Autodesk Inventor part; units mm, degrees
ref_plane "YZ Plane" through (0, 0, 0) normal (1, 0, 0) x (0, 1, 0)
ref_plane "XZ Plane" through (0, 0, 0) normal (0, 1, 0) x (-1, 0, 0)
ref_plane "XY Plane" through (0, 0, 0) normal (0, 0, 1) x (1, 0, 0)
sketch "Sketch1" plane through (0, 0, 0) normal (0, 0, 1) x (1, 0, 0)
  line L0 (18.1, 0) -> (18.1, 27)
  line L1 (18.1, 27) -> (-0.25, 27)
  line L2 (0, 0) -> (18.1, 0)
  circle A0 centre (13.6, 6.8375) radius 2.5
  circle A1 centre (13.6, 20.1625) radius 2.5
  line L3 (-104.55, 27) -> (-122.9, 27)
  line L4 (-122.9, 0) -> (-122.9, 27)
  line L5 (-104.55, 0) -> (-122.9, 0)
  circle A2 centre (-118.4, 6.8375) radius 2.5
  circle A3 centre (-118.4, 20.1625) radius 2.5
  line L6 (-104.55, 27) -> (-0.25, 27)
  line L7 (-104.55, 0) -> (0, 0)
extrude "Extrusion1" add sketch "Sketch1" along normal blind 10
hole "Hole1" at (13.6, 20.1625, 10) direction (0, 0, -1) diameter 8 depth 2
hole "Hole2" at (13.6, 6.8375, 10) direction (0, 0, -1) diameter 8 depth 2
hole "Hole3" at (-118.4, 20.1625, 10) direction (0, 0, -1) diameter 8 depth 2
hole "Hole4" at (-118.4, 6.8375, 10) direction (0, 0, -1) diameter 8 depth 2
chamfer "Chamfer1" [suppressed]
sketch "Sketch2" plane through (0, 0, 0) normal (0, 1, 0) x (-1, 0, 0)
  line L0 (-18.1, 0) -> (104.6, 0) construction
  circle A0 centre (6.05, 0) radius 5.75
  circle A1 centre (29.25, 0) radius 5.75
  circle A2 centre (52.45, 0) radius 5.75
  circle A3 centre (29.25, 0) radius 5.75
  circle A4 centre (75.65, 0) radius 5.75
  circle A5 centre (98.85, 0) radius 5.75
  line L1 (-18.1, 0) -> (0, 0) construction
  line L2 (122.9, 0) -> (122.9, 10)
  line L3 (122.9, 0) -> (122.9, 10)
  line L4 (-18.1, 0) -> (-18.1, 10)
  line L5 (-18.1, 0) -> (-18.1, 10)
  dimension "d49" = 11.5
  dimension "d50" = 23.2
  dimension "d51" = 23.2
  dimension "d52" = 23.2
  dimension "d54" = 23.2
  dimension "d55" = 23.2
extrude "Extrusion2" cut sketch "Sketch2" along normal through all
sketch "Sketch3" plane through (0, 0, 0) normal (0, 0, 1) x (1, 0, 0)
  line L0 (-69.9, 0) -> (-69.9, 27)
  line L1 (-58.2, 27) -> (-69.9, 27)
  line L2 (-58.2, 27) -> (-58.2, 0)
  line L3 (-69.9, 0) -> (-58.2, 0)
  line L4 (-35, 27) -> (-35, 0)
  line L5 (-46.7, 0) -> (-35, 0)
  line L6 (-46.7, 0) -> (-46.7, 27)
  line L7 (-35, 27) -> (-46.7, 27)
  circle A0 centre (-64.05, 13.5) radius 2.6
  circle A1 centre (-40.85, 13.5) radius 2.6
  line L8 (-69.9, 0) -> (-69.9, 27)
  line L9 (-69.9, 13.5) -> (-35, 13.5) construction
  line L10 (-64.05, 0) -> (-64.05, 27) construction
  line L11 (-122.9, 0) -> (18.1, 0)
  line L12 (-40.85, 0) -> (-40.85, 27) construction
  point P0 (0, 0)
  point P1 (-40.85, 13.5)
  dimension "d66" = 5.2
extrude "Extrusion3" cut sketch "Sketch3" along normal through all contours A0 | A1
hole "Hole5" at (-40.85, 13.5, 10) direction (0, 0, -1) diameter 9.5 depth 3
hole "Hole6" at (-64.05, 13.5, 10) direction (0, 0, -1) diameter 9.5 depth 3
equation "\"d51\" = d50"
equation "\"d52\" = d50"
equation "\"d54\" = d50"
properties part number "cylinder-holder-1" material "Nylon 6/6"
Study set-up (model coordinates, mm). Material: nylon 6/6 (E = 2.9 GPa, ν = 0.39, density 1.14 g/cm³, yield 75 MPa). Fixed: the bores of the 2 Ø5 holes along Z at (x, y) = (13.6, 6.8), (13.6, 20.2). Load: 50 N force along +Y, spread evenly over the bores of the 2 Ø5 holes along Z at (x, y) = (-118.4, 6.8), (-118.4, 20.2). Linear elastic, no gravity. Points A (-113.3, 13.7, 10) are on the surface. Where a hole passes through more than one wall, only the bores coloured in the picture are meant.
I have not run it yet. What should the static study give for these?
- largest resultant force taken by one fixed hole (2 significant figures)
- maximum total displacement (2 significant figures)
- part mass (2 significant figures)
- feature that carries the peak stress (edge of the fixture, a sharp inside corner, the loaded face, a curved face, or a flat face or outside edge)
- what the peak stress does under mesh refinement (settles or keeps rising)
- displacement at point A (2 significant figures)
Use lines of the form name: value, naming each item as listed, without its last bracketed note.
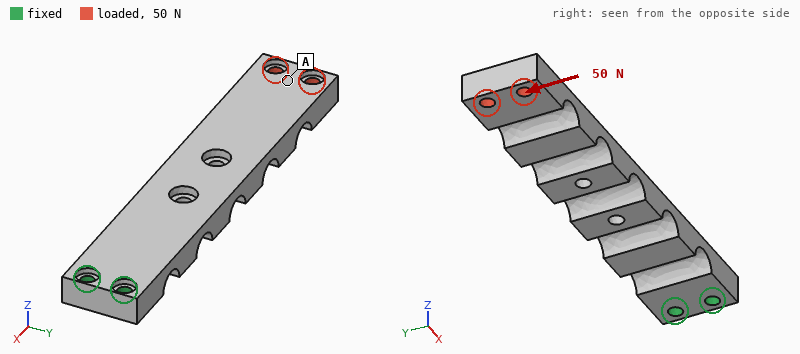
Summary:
largest resultant force taken by one fixed hole: 390 N
maximum total displacement: 1.7 mm
part mass: 33 g
feature that carries the peak stress: edge of the fixture
what the peak stress does under mesh refinement: keeps rising
displacement at point A: 1.4 mm
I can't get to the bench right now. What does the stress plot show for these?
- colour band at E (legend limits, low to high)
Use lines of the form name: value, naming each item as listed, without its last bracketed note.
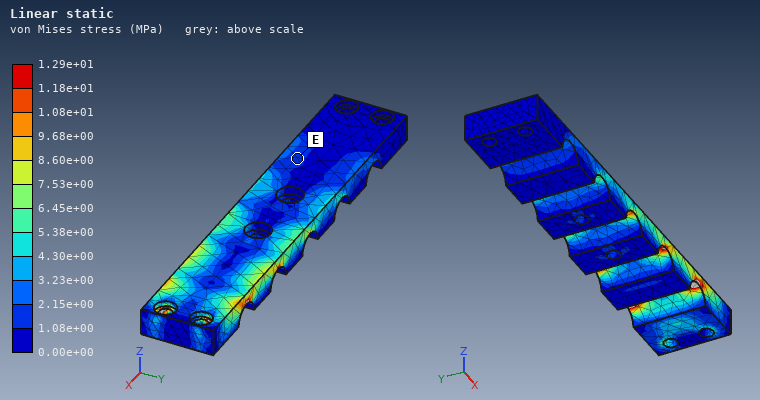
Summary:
colour band at E: 1.08e+00 to 2.15e+00 MPa
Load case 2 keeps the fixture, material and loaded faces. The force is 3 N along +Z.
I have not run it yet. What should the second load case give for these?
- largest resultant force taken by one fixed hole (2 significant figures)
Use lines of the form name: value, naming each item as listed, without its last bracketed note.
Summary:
largest resultant force taken by one fixed hole: 1.7 N
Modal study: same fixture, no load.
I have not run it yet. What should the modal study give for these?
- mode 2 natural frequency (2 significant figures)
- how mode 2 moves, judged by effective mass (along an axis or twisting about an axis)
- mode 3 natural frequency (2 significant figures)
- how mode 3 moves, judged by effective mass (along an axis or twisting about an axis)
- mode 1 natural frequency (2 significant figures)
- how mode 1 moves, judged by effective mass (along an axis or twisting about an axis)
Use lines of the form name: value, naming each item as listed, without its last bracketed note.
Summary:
mode 2 natural frequency: 300 Hz
how mode 2 moves, judged by effective mass: along Y
mode 3 natural frequency: 480 Hz
how mode 3 moves, judged by effective mass: along Z
mode 1 natural frequency: 76 Hz
how mode 1 moves, judged by effective mass: along Z
